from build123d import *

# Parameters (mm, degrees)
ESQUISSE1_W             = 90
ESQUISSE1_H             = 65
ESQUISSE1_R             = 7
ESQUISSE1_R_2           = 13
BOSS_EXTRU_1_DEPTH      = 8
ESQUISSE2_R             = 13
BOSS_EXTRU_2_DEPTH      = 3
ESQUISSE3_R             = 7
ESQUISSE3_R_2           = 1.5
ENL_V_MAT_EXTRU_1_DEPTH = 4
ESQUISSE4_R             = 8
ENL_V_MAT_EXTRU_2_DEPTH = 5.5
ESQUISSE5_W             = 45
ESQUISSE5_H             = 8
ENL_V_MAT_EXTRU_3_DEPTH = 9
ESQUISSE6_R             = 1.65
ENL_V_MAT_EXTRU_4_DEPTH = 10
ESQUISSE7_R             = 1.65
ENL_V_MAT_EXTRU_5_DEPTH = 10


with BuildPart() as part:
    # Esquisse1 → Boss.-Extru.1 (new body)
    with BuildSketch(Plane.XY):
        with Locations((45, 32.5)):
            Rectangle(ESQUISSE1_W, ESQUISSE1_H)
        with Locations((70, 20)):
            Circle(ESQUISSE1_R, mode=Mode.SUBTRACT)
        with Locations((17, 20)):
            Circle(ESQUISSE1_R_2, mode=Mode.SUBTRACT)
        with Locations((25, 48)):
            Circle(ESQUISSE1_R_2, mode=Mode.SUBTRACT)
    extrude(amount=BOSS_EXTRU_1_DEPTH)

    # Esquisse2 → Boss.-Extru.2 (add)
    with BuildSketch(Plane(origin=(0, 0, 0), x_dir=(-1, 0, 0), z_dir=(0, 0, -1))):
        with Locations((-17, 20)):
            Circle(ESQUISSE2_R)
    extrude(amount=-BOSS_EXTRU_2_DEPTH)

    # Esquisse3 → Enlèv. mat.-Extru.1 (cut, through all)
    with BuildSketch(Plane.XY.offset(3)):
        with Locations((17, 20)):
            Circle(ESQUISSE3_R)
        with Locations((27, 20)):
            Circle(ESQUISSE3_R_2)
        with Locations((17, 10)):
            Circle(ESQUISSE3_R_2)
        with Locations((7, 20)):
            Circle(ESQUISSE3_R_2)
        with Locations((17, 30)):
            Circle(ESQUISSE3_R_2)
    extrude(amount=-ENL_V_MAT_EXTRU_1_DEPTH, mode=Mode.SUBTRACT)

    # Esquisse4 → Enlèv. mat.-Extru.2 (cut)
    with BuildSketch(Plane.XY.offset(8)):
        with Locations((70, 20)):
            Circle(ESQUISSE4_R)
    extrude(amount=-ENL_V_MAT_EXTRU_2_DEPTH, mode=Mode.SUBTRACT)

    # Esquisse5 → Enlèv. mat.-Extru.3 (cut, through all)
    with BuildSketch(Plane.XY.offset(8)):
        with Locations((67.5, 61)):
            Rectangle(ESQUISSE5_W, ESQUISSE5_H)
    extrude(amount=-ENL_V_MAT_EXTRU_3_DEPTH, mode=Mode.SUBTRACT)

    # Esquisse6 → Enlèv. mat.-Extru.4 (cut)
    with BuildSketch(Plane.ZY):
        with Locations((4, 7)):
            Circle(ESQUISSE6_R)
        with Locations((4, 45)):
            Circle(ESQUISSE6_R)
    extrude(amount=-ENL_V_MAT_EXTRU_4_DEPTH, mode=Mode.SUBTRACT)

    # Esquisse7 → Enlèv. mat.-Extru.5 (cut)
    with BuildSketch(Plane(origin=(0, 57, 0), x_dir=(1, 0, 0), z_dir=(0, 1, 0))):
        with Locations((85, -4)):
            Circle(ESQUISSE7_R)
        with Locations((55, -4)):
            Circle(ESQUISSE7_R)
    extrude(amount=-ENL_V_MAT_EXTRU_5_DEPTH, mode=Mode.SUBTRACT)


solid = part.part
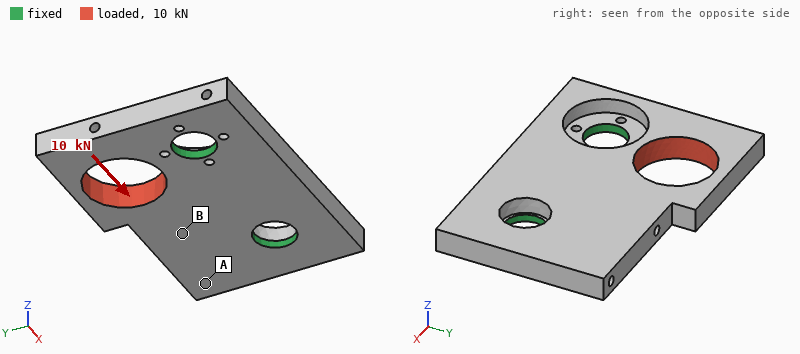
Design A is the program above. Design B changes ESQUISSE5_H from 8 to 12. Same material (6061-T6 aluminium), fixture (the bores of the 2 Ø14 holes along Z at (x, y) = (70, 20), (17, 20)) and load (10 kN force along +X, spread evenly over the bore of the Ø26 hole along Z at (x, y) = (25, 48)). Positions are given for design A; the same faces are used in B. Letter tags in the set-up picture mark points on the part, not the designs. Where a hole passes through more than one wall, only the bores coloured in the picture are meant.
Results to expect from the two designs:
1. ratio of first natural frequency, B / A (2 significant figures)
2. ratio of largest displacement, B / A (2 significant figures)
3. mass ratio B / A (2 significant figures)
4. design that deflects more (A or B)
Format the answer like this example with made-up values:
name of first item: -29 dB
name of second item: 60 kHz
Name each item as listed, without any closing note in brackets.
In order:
ratio of first natural frequency, B / A: 1.0
ratio of largest displacement, B / A: 1.1
mass ratio B / A: 0.98
design that deflects more: B
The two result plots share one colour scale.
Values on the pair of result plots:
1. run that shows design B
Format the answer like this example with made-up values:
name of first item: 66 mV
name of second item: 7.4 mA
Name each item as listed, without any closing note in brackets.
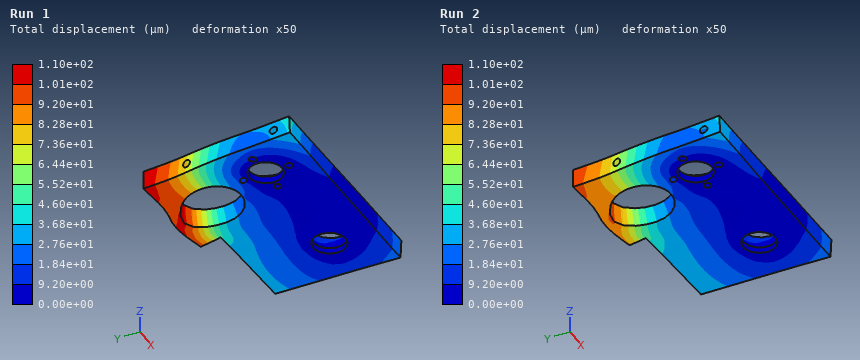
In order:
run that shows design B: Run 1
